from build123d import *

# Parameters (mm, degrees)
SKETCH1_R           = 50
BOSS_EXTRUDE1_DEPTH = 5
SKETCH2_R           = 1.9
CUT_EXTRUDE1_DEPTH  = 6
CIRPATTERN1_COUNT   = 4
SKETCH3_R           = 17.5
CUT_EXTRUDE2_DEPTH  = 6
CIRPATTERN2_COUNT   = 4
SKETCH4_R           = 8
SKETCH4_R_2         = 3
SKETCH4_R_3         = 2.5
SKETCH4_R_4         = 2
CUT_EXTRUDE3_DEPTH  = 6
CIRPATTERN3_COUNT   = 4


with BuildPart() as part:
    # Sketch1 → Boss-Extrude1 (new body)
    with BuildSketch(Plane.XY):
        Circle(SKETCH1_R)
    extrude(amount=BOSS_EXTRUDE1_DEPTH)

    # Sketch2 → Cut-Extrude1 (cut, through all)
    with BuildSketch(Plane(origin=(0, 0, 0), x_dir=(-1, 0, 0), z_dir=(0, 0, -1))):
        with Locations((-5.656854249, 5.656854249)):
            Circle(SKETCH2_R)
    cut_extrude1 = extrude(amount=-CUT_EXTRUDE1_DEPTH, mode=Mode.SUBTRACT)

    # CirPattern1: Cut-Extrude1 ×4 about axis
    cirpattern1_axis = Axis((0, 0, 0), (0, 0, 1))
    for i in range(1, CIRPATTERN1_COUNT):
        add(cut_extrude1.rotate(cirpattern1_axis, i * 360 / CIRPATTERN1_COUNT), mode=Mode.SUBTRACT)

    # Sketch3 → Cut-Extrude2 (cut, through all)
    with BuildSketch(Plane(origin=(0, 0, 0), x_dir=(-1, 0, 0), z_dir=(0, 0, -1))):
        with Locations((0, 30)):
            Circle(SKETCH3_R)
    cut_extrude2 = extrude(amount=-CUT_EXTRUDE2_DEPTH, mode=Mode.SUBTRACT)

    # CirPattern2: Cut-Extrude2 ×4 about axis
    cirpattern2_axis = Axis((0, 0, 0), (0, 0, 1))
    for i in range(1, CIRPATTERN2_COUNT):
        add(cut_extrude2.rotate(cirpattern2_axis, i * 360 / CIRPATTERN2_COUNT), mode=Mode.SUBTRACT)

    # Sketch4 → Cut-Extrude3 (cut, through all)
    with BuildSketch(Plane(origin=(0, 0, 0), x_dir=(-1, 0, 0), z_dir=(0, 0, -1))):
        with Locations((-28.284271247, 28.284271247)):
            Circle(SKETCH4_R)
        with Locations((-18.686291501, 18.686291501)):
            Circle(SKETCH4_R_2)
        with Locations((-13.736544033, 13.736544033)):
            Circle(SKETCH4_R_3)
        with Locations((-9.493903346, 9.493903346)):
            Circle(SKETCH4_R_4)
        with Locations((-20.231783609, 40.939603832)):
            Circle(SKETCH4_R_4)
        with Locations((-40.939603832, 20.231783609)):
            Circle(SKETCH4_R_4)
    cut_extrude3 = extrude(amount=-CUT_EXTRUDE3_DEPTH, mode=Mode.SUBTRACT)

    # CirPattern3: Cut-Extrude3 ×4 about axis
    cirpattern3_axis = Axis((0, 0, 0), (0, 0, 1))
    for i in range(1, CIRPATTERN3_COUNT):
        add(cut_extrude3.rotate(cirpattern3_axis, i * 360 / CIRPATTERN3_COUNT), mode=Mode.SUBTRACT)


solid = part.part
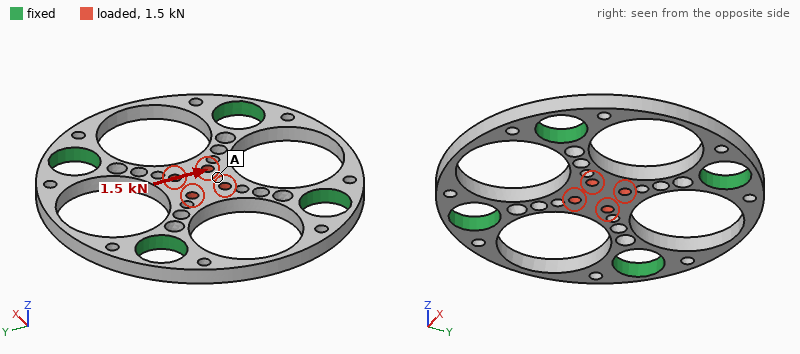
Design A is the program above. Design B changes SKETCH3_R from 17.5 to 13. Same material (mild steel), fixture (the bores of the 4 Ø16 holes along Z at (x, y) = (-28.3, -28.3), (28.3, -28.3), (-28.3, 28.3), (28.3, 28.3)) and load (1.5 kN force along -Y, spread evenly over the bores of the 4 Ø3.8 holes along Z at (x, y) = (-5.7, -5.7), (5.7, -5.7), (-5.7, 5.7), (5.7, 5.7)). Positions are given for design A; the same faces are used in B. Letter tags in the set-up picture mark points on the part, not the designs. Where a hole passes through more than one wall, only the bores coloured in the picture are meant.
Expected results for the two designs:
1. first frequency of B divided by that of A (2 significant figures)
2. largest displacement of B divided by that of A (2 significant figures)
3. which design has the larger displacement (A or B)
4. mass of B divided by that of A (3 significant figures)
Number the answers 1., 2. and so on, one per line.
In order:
1. 1.2
2. 0.36
3. A
4. 1.61
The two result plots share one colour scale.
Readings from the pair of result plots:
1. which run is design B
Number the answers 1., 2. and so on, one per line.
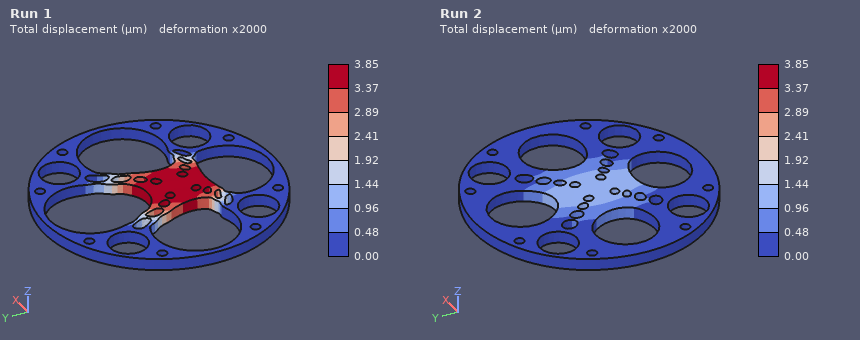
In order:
1. Run 2
